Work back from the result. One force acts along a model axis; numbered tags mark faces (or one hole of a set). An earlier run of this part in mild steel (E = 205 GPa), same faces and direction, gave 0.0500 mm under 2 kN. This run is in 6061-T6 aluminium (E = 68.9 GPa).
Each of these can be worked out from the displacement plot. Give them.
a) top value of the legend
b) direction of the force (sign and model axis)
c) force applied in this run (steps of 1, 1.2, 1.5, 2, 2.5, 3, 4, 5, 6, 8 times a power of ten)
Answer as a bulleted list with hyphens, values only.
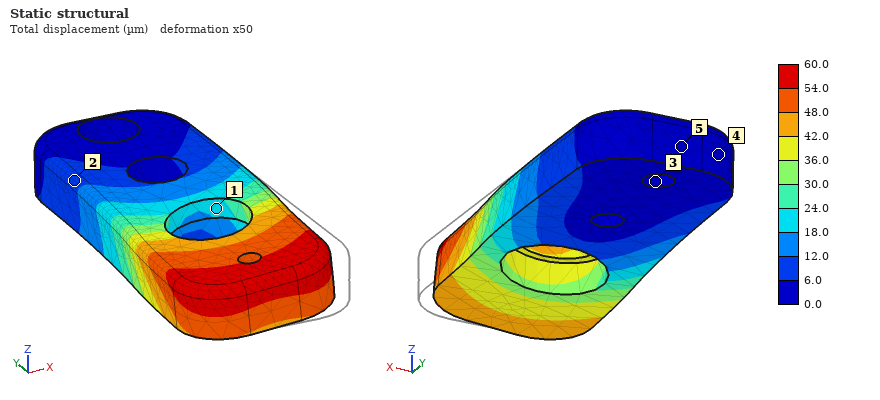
- 60.0 µm
- -X
- 800 N
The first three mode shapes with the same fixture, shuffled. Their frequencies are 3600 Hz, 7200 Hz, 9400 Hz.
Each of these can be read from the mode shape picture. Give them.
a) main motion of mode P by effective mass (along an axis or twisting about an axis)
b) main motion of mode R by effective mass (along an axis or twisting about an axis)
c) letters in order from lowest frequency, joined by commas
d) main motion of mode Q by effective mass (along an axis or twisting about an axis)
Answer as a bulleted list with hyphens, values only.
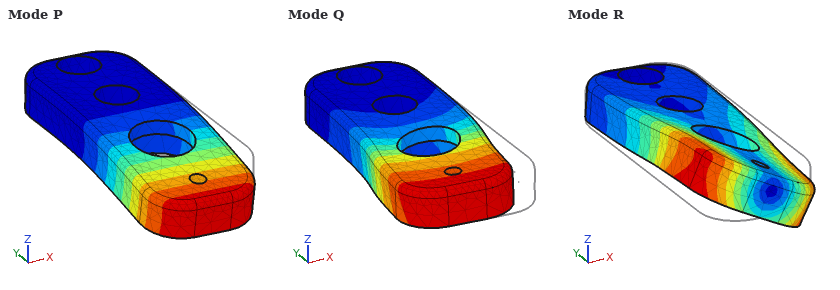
- along Z
- twisting about Y
- P, Q, R
- along X
